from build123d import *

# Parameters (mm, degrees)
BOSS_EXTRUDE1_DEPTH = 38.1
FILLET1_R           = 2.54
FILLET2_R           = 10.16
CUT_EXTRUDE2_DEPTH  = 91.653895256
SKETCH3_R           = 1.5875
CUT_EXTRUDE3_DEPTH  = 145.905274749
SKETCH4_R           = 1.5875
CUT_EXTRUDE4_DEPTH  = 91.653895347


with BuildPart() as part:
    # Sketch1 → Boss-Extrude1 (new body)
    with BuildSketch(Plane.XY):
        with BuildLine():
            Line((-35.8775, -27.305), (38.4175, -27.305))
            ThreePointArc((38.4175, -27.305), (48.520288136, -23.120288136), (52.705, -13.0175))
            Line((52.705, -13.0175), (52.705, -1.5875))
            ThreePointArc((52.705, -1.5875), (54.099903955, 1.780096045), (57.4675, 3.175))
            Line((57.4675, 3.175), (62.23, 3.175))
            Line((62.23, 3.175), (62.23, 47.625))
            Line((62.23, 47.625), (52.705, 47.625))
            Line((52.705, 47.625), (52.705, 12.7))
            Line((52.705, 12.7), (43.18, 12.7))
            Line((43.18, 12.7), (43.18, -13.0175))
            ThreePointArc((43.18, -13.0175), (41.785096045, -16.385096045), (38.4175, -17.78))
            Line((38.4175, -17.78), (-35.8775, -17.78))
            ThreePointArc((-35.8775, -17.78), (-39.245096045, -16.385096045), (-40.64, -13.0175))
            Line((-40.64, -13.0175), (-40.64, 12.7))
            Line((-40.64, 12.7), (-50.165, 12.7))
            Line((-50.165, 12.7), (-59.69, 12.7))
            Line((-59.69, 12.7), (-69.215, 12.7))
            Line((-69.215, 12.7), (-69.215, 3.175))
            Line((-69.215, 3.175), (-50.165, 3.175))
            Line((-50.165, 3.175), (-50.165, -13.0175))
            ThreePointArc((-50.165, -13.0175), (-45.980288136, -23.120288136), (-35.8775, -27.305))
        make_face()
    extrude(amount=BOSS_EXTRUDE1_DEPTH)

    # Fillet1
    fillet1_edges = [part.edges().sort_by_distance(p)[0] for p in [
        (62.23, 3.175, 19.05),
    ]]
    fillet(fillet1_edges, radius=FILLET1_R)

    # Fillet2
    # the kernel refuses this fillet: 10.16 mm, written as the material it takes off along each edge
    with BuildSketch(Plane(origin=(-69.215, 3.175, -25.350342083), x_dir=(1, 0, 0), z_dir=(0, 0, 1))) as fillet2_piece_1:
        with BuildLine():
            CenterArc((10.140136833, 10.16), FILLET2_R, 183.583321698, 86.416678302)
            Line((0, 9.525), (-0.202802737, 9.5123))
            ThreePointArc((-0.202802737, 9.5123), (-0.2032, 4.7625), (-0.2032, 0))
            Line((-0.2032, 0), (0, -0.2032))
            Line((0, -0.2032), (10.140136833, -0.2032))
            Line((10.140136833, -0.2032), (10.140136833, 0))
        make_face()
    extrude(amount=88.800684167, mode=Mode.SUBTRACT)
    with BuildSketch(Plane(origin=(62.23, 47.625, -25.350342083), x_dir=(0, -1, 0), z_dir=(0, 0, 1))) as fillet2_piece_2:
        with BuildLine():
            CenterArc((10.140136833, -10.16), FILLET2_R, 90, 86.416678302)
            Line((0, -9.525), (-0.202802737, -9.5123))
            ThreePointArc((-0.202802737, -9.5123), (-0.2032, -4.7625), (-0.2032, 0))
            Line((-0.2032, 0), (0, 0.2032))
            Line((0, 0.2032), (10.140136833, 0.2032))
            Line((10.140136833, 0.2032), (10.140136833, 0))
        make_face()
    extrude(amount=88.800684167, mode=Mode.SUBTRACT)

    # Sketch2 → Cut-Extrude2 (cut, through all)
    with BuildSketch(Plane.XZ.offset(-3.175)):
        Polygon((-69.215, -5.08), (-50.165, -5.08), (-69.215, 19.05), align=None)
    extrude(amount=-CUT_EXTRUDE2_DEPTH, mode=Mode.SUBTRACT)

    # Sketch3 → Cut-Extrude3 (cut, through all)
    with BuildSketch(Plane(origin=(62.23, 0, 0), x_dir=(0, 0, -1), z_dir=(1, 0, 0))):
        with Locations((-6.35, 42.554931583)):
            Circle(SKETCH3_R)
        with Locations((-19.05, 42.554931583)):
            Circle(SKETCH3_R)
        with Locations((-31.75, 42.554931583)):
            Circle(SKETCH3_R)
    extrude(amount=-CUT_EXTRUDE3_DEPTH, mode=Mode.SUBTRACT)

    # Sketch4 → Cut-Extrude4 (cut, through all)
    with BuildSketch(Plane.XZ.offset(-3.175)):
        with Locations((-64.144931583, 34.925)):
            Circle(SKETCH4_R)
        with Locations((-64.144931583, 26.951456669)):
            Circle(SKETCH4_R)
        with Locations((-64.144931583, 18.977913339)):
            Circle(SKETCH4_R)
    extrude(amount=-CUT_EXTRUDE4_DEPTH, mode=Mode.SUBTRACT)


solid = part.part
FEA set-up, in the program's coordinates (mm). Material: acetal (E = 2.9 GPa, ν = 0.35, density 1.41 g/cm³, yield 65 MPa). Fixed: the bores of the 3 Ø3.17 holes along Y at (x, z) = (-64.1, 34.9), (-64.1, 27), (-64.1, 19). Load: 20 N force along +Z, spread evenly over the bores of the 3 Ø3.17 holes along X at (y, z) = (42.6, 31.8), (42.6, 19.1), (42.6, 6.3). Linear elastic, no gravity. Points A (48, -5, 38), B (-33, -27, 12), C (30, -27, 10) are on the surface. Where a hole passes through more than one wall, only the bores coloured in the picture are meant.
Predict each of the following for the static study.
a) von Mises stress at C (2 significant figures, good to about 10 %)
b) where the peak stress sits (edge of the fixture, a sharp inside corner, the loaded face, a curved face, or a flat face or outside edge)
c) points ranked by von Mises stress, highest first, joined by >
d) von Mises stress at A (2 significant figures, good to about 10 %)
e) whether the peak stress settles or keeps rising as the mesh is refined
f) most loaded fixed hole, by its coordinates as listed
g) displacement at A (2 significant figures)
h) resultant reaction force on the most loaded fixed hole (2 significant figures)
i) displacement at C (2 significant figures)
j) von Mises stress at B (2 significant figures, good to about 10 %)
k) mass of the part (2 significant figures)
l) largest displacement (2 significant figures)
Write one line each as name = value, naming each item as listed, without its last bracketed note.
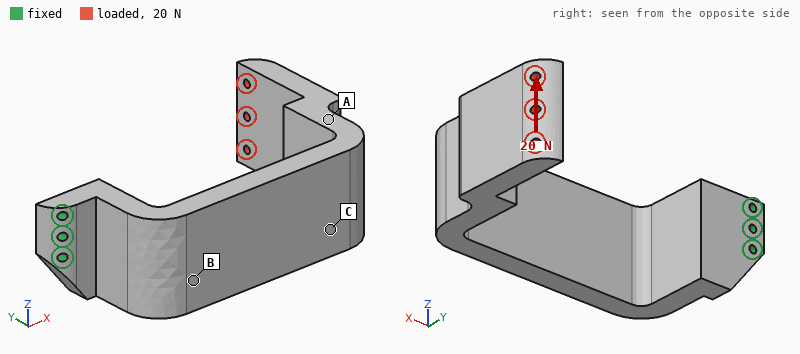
von Mises stress at C = 1.9 MPa
where the peak stress sits = edge of the fixture
points ranked by von Mises stress, highest first, joined by > = B > C > A
von Mises stress at A = 0.45 MPa
whether the peak stress settles or keeps rising as the mesh is refined = keeps rising
most loaded fixed hole, by its coordinates as listed = (-64.1, 19)
displacement at A = 0.86 mm
resultant reaction force on the most loaded fixed hole = 150 N
displacement at C = 0.43 mm
von Mises stress at B = 2.5 MPa
mass of the part = 110 g
largest displacement = 1.7 mm
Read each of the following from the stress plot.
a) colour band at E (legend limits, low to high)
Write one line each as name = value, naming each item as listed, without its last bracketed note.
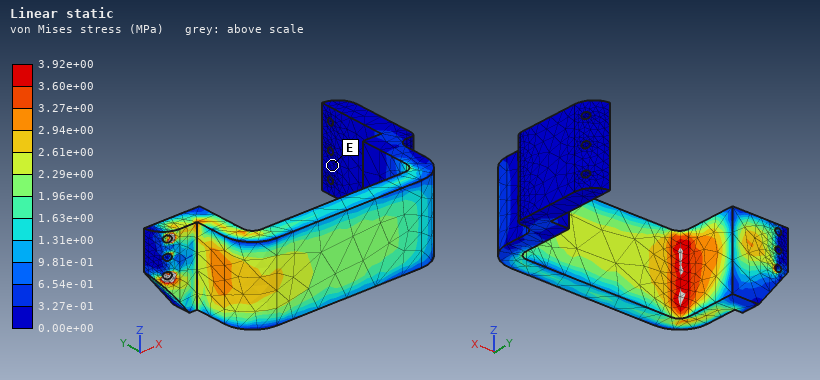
colour band at E = 0.00e+00 to 3.27e-01 MPa
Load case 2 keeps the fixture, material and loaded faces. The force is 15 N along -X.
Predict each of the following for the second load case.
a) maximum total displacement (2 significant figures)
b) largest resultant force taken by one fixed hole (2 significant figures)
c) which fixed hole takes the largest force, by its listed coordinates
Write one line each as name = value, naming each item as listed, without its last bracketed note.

maximum total displacement = 1.5 mm
largest resultant force taken by one fixed hole = 13 N
which fixed hole takes the largest force, by its listed coordinates = (-64.1, 19)
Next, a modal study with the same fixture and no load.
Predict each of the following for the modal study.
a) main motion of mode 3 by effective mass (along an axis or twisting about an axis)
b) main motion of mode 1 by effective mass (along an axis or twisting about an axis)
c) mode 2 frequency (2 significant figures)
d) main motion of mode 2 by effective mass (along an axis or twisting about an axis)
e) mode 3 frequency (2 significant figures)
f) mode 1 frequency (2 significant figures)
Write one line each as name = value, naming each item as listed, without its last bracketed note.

main motion of mode 3 by effective mass = along X
main motion of mode 1 by effective mass = along Y
mode 2 frequency = 110 Hz
main motion of mode 2 by effective mass = along Z
mode 3 frequency = 230 Hz
mode 1 frequency = 66 Hz
